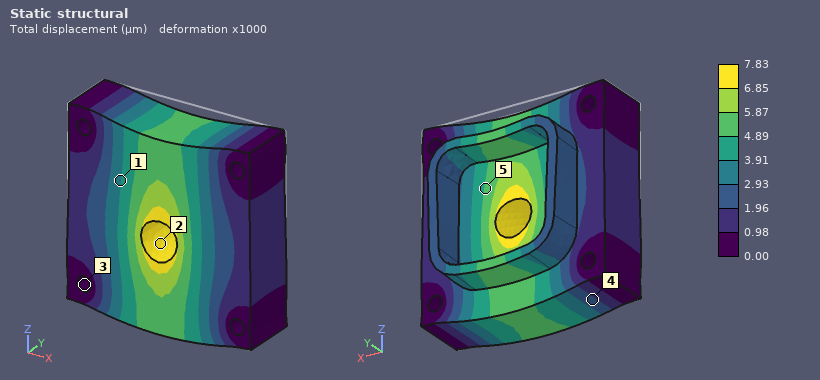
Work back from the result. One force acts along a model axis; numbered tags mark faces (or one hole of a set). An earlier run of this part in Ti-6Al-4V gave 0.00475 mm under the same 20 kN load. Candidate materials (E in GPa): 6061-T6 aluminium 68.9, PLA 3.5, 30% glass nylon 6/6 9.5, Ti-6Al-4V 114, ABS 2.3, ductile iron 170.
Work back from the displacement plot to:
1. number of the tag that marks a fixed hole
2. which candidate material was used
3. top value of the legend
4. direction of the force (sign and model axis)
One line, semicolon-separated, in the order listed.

3; 6061-T6 aluminium; 7.83 µm; -Z
